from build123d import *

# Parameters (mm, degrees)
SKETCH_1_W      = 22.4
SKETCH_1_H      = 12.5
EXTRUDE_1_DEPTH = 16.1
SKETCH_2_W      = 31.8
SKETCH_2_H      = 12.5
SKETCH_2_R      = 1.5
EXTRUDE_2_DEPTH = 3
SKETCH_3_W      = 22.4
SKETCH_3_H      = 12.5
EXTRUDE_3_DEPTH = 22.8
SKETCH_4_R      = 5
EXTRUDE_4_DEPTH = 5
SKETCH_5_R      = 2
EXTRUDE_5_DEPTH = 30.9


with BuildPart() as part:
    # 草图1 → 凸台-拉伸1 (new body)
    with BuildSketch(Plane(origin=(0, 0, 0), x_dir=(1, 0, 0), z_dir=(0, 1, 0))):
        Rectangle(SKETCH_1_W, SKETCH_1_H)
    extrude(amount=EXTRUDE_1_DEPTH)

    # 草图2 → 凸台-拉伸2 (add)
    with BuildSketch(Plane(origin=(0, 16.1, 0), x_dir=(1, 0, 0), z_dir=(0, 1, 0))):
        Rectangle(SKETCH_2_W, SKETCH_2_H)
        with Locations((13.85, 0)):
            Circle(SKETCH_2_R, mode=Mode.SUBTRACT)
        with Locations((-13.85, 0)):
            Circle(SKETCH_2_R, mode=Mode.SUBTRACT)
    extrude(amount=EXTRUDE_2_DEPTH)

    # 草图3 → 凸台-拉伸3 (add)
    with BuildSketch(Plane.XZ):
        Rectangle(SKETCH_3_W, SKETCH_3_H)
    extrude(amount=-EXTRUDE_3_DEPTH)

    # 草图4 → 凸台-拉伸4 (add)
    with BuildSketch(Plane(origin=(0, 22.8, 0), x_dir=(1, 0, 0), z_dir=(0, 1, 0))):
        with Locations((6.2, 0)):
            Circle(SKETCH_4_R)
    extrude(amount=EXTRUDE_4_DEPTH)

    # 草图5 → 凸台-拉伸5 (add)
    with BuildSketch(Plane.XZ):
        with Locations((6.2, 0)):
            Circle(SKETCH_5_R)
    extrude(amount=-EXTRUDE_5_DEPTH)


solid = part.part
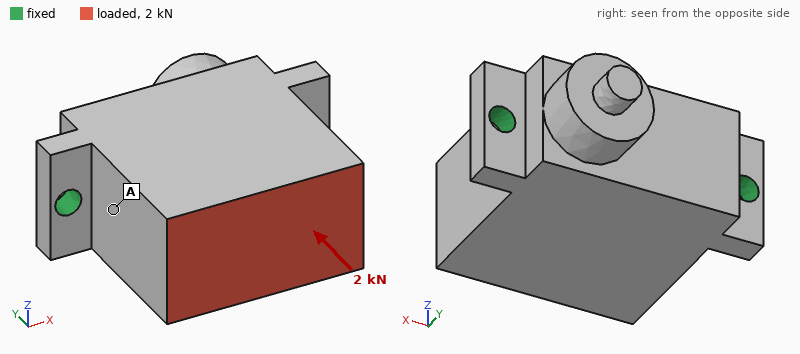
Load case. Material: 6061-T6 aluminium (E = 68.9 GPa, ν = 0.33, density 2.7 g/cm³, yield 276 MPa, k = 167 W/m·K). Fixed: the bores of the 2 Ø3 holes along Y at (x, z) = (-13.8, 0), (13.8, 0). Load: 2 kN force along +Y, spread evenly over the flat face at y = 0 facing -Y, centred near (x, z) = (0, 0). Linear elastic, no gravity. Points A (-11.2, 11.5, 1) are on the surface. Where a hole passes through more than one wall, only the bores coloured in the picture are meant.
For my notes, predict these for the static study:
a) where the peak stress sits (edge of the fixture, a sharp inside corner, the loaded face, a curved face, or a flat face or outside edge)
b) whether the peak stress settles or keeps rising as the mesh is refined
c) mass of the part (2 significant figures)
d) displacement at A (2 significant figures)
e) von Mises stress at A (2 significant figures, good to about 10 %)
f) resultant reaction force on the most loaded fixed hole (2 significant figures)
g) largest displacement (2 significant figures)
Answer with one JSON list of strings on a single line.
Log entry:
["edge of the fixture", "keeps rising", "19 g", "7.6 µm", "18 MPa", "1.0 kN", "9.2 µm"]
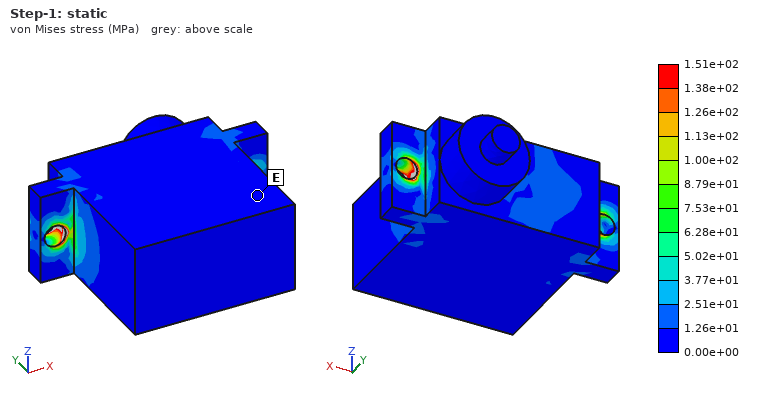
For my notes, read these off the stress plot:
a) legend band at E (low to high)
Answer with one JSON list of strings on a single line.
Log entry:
["0.00e+00 to 1.26e+01 MPa"]
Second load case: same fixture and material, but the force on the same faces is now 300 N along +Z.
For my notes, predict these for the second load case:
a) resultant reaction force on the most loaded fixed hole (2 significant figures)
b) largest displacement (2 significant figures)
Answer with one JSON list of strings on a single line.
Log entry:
["150 N", "52 µm"]
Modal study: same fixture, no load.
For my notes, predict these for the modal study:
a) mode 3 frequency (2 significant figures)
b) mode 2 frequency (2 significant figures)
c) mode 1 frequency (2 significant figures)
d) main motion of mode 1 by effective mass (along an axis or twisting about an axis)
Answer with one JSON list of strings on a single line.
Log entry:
["19 kHz", "19 kHz", "5300 Hz", "along Z"]
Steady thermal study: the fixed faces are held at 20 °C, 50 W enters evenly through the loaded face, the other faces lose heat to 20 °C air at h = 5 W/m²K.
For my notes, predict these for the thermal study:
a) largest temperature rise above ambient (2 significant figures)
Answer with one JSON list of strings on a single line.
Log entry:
["37 K"]
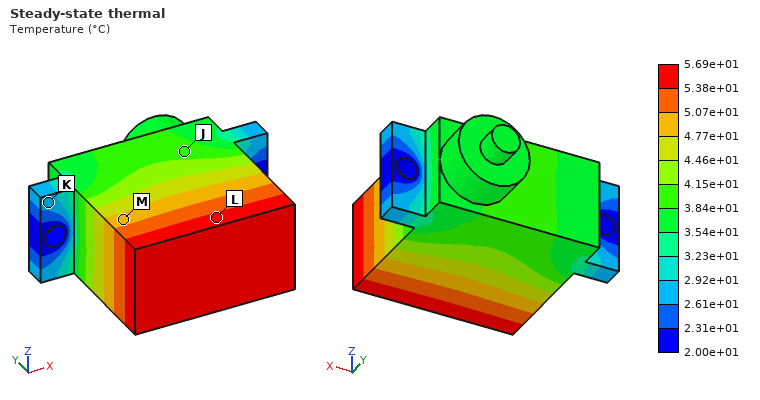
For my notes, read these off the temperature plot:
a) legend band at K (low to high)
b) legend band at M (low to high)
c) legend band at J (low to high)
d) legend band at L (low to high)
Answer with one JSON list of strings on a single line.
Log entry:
["2.61e+01 to 2.92e+01 °C", "4.77e+01 to 5.07e+01 °C", "3.84e+01 to 4.15e+01 °C", "5.38e+01 to 5.69e+01 °C"]
